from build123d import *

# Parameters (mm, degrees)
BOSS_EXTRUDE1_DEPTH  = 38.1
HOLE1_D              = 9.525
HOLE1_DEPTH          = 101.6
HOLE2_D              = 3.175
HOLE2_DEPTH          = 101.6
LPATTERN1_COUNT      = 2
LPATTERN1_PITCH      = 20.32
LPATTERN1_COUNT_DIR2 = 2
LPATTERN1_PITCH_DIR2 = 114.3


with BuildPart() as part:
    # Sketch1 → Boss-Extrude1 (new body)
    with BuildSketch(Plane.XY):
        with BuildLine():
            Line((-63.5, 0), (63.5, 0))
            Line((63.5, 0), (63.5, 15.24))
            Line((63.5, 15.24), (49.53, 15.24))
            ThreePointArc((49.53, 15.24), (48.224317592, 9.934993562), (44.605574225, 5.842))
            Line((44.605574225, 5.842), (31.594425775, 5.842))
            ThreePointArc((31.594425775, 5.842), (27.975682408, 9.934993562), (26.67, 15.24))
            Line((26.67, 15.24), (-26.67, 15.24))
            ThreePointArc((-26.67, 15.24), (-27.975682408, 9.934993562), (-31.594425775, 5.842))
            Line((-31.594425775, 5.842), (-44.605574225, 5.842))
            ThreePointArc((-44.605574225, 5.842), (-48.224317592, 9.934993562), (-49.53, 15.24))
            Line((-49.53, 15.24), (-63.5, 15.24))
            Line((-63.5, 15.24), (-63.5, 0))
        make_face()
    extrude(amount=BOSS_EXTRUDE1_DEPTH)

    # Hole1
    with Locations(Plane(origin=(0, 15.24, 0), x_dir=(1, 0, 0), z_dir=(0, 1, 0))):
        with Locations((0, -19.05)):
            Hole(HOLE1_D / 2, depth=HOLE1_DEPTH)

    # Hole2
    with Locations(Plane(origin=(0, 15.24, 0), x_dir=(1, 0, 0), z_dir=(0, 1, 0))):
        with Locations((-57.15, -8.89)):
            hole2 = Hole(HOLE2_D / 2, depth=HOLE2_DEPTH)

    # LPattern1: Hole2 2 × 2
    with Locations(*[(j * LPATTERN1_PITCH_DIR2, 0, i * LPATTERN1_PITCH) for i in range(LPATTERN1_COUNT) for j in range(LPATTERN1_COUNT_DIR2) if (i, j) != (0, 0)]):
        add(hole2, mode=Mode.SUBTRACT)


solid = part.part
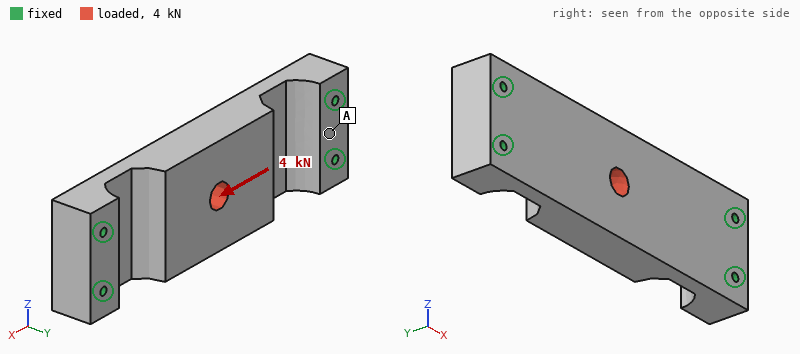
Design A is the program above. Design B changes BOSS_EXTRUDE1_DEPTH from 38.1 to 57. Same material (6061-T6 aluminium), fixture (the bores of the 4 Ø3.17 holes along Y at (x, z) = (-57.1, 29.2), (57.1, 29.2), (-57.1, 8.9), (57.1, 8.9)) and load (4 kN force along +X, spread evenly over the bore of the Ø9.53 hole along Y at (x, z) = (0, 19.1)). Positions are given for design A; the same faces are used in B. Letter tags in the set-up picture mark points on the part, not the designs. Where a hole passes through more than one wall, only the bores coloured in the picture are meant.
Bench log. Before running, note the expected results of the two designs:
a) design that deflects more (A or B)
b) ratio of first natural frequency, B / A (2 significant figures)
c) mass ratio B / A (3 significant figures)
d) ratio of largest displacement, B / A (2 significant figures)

A
0.88
1.51
0.92
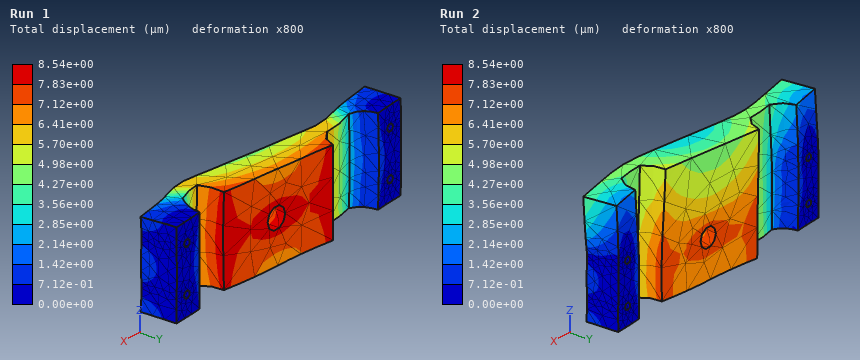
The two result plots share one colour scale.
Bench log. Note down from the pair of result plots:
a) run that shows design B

Run 2
